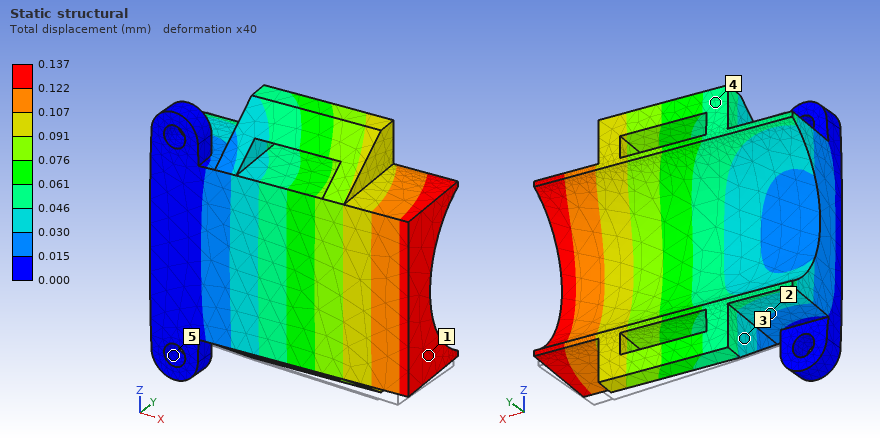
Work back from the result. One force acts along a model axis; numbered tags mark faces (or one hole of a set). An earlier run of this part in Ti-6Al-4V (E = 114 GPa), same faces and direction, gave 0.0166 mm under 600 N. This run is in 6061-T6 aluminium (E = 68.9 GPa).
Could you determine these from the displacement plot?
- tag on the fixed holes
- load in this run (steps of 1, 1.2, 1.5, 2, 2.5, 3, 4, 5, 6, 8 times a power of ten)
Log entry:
5
3 kN
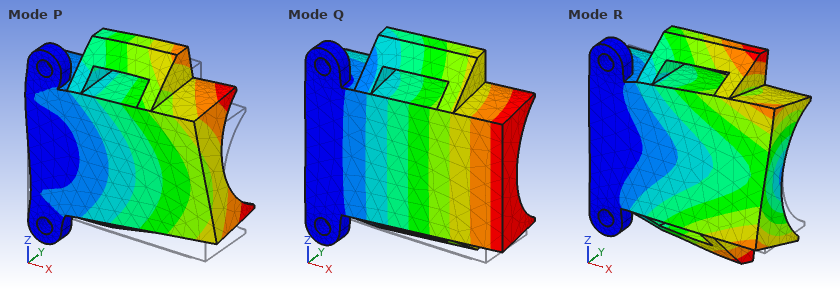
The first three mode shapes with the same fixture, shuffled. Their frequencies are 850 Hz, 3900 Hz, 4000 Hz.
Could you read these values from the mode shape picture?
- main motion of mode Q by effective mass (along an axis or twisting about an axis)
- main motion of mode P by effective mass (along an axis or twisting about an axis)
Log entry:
along Y
along Z
